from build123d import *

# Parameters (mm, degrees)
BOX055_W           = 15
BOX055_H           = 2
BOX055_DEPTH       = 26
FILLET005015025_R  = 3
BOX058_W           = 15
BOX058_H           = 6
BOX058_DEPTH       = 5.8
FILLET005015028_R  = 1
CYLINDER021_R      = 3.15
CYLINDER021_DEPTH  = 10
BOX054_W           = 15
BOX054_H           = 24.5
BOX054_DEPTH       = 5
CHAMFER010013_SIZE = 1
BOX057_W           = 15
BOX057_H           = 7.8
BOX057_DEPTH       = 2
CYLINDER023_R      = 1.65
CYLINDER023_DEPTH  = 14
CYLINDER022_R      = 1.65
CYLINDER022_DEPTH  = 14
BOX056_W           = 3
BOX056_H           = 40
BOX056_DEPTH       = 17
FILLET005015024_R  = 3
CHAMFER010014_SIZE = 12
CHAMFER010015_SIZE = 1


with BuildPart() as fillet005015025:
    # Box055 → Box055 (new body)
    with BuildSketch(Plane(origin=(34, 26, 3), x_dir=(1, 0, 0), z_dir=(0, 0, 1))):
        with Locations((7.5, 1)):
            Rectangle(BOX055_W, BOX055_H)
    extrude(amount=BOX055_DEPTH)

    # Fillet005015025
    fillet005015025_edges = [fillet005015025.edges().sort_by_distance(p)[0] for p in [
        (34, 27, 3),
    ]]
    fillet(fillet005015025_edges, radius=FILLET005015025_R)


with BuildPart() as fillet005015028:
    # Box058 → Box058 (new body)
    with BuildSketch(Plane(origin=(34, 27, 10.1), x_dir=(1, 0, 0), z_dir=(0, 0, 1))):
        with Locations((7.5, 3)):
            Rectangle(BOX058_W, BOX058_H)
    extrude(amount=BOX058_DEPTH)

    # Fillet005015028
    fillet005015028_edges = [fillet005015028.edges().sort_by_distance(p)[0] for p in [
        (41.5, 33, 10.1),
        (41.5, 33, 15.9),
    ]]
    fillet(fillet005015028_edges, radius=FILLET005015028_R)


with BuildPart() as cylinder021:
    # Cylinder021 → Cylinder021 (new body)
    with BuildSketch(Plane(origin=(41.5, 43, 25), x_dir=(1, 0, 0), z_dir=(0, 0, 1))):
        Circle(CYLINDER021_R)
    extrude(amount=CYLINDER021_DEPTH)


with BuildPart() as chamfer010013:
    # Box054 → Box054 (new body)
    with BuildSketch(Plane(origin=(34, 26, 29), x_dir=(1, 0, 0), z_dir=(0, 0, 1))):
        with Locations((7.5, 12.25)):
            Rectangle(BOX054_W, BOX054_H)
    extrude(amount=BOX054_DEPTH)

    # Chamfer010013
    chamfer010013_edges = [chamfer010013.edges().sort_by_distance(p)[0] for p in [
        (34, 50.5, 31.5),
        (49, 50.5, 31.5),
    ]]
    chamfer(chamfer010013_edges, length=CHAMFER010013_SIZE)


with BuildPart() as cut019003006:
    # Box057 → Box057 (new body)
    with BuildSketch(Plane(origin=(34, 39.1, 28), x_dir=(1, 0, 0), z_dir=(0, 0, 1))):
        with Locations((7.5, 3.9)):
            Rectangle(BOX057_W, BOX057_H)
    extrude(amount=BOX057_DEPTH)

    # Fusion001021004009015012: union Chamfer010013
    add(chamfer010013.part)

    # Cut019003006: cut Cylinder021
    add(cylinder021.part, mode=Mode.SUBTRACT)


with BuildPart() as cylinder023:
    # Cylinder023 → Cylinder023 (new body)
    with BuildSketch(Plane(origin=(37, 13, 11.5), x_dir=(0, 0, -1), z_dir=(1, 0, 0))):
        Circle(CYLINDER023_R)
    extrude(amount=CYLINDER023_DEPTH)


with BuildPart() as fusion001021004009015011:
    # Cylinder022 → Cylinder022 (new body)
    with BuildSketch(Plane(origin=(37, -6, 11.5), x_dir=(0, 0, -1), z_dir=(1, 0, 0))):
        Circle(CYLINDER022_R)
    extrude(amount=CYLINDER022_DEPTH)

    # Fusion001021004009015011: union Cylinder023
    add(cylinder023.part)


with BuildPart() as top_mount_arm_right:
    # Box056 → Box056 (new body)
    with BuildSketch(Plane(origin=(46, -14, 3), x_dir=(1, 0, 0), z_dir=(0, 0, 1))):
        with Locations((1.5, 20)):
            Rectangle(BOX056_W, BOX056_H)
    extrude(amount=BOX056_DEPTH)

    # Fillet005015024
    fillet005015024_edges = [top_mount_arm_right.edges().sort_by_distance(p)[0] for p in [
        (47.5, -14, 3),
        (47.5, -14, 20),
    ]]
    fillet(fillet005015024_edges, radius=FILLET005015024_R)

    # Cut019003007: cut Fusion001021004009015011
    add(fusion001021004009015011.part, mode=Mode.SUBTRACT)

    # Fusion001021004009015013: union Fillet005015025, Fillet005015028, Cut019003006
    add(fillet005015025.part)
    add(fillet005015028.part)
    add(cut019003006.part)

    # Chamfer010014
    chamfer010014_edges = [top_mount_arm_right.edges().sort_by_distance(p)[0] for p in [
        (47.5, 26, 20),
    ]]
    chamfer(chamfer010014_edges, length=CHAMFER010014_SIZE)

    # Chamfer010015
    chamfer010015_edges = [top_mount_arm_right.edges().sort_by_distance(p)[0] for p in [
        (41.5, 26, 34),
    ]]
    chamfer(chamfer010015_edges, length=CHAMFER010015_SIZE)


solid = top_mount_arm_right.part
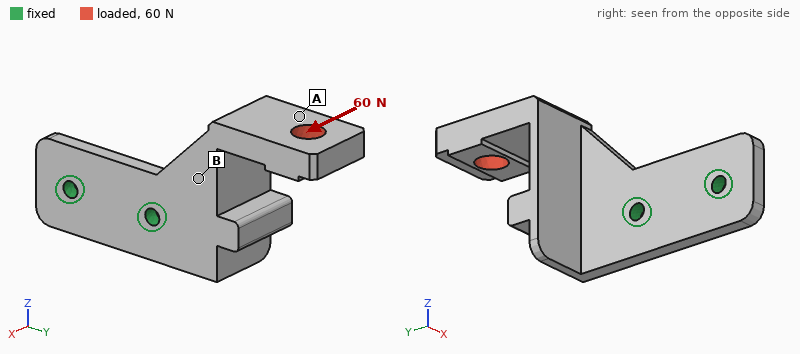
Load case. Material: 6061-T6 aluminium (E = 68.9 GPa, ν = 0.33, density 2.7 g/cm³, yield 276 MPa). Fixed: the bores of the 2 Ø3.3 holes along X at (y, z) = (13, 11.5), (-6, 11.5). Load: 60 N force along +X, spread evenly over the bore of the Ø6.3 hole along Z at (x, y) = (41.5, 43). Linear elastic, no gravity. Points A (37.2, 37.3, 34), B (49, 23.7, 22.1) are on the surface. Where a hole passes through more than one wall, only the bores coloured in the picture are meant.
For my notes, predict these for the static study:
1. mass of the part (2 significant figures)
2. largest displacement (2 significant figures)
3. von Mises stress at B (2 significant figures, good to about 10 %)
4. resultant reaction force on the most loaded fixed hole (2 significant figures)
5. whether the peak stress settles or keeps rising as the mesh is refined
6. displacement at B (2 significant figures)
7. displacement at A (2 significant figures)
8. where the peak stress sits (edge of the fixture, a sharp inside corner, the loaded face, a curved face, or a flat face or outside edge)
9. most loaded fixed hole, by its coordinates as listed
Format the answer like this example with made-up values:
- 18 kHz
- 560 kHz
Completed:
- 14 g
- 0.43 mm
- 40 MPa
- 81 N
- keeps rising
- 0.069 mm
- 0.28 mm
- edge of the fixture
- (13, 11.5)
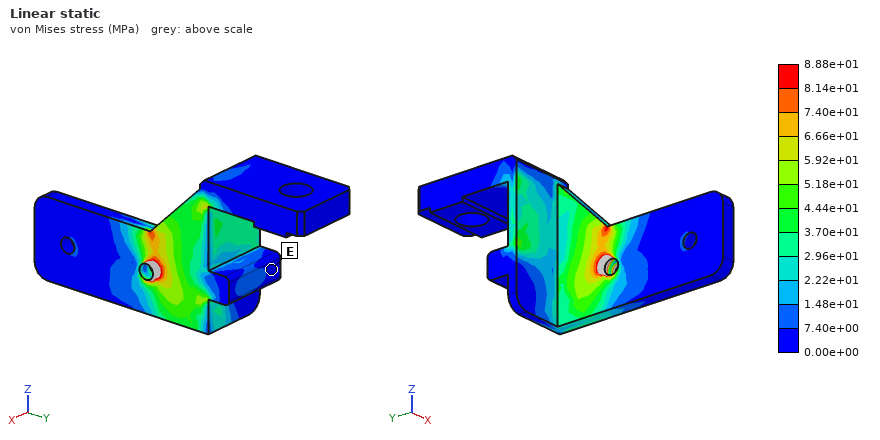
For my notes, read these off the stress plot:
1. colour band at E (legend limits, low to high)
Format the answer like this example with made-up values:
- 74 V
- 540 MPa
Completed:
- 0.00e+00 to 7.40e+00 MPa
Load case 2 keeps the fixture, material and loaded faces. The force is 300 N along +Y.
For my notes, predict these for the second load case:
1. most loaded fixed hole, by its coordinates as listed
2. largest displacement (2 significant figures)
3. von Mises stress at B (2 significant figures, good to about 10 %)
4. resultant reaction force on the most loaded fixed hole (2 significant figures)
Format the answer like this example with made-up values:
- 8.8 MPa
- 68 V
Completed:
- (13, 11.5)
- 0.52 mm
- 60 MPa
- 320 N
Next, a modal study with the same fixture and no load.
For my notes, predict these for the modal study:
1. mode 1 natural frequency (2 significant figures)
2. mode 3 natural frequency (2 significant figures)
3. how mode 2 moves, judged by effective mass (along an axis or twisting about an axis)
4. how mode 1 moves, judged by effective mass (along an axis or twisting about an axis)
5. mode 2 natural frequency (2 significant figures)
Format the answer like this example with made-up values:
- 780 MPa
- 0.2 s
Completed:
- 1100 Hz
- 3900 Hz
- along Z
- along X
- 2300 Hz
